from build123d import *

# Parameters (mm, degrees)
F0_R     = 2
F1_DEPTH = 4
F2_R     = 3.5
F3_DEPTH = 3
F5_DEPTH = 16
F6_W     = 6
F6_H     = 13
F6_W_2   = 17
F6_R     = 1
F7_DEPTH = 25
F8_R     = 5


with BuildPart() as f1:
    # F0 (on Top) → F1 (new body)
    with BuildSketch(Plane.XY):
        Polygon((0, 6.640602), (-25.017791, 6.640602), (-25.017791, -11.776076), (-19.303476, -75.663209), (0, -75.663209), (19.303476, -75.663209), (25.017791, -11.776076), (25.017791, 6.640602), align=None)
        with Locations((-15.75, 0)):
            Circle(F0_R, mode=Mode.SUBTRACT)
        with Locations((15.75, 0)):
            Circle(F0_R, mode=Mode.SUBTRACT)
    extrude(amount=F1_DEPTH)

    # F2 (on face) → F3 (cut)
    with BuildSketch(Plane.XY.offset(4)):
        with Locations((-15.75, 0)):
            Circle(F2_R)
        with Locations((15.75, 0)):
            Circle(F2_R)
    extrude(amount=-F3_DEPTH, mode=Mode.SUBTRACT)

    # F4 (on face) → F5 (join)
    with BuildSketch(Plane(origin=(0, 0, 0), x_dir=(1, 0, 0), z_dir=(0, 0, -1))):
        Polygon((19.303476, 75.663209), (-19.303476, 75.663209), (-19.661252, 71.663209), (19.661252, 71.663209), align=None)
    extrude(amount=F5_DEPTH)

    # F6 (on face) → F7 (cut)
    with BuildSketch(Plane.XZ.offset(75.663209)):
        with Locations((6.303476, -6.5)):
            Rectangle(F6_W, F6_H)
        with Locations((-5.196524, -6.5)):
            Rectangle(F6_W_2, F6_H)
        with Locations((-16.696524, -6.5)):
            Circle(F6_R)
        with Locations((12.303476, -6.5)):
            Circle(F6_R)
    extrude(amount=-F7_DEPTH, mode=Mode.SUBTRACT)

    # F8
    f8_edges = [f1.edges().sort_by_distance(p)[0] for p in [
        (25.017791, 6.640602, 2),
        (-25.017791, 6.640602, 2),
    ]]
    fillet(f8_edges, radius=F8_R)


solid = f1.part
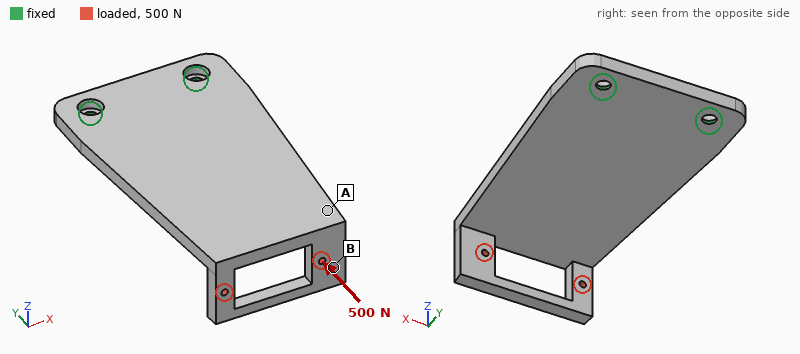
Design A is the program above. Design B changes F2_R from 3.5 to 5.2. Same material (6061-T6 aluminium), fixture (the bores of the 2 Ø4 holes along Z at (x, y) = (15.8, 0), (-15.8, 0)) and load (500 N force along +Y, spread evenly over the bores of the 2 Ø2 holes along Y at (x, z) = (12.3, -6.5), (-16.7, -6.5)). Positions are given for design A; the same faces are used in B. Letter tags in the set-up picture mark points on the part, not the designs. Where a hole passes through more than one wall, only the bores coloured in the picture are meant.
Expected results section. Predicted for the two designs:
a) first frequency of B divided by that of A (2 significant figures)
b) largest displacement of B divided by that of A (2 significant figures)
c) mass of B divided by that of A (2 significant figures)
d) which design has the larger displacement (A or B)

0.83
1.3
0.98
B
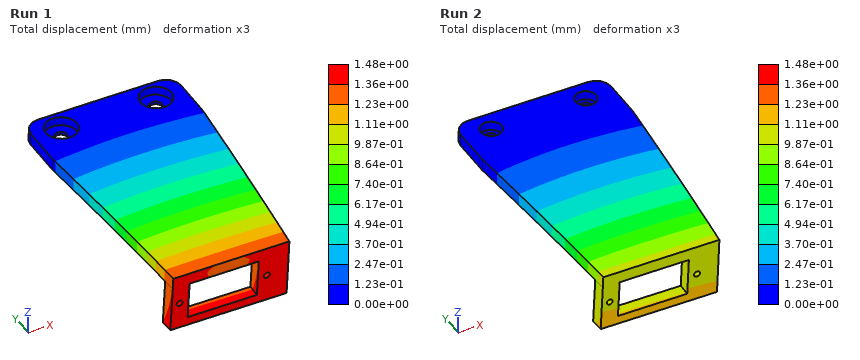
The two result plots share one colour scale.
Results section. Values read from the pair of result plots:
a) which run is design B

Run 1
